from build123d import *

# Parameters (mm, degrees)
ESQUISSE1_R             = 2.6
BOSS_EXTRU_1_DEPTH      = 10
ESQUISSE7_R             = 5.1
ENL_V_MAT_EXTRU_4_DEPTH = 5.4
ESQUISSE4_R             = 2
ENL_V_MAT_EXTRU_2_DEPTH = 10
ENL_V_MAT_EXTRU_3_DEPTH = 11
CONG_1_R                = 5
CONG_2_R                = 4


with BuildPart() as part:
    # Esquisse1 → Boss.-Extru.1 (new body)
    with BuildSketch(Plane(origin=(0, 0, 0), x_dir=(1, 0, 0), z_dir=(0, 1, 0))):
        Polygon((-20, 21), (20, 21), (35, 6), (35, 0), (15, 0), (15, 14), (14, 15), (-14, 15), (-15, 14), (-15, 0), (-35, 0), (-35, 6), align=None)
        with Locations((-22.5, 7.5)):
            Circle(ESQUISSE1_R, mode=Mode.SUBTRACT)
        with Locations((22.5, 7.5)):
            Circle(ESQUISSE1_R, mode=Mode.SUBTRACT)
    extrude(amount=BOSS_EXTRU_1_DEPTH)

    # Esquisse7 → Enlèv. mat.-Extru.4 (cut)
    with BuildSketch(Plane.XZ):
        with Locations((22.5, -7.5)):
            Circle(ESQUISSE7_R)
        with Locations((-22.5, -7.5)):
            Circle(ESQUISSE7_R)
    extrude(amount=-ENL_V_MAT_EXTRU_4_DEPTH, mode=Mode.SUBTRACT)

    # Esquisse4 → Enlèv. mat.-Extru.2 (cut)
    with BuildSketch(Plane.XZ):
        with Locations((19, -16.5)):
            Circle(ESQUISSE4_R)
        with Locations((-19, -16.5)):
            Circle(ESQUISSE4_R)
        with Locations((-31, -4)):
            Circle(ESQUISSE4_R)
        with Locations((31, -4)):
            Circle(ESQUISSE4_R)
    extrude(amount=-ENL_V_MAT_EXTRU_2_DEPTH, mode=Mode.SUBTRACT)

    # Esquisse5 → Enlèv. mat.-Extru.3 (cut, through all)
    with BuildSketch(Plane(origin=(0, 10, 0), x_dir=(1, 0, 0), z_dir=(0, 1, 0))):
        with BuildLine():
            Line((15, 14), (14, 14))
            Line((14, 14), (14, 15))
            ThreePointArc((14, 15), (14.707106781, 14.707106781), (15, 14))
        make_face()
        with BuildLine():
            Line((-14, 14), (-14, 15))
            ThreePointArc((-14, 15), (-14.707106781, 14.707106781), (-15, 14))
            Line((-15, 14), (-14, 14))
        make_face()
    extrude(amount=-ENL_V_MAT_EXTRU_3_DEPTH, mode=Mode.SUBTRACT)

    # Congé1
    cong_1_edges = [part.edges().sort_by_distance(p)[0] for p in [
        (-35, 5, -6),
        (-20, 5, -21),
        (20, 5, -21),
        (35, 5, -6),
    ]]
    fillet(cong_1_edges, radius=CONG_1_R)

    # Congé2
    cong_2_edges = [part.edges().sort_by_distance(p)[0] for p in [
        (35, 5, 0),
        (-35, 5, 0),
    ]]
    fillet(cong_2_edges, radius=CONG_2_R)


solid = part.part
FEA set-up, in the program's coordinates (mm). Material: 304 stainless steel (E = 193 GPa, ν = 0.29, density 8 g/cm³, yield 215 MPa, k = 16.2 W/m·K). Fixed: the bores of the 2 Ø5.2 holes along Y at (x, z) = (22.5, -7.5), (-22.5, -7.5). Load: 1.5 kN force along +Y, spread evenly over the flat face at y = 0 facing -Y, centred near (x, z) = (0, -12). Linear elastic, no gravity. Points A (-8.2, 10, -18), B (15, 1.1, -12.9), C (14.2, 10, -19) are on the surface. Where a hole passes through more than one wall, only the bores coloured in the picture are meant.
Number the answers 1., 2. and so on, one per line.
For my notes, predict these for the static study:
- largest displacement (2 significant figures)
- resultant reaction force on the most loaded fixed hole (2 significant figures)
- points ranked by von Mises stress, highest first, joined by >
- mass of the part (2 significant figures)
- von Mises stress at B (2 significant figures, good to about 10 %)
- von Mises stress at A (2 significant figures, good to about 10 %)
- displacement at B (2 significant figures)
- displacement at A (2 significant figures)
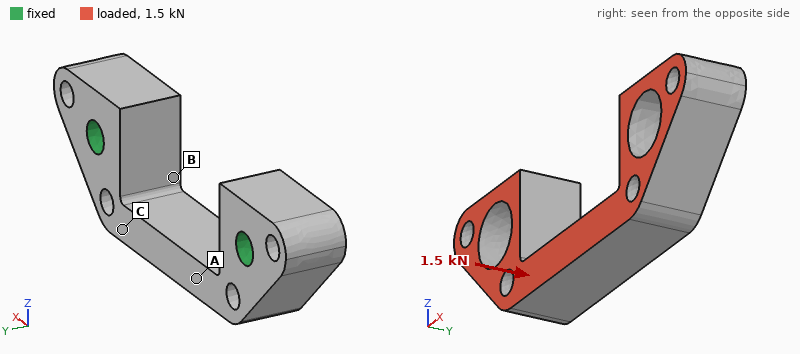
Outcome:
1. 8.3 µm
2. 750 N
3. B > A > C
4. 50 g
5. 20 MPa
6. 13 MPa
7. 3.4 µm
8. 6.0 µm
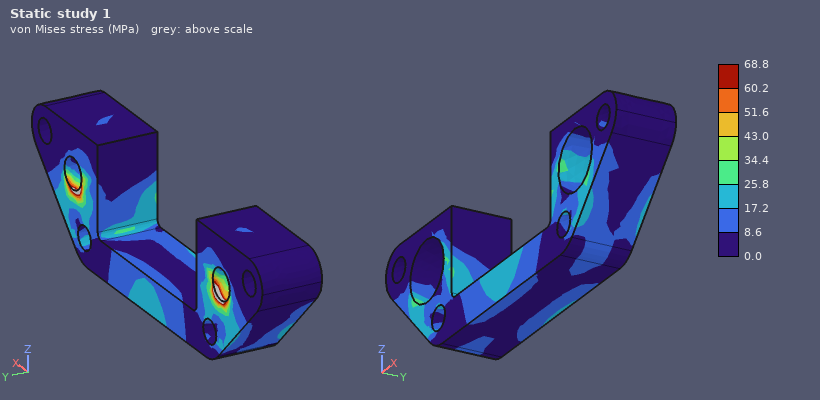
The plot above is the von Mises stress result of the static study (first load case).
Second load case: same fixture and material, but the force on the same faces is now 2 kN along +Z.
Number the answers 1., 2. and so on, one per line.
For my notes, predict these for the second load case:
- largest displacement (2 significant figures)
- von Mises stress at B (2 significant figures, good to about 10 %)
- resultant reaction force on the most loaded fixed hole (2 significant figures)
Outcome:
1. 16 µm
2. 52 MPa
3. 1.0 kN
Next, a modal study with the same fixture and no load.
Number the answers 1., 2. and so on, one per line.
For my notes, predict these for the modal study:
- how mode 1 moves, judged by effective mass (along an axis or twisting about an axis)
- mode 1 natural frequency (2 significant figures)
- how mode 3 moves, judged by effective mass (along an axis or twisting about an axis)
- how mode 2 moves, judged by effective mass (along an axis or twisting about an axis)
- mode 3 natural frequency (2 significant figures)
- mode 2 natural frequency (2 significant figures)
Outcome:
1. along Y
2. 11 kHz
3. along X
4. along Z
5. 19 kHz
6. 18 kHz
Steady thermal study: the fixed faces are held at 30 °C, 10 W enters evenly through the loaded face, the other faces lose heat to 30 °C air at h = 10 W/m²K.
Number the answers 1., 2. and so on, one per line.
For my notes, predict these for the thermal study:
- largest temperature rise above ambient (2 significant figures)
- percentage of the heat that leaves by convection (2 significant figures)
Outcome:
1. 43 K
2. 6.4 %
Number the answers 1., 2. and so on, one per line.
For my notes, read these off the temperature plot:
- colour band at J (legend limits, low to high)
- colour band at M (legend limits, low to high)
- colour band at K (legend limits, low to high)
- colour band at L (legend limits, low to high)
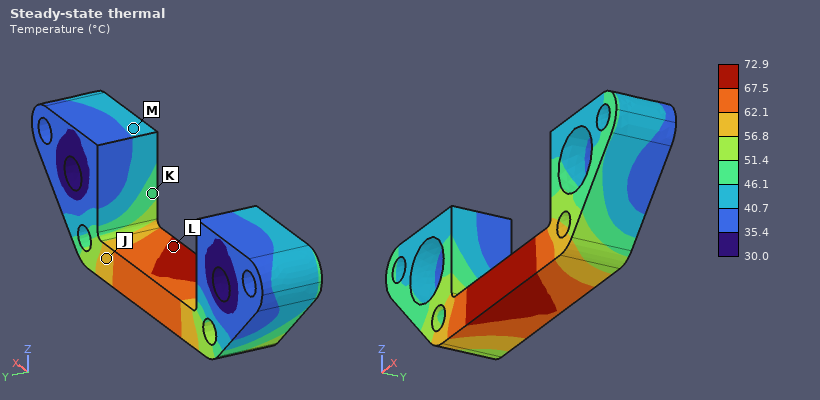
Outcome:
1. 56.8 to 62.1 °C
2. 40.7 to 46.1 °C
3. 46.1 to 51.4 °C
4. 67.5 to 72.9 °C
